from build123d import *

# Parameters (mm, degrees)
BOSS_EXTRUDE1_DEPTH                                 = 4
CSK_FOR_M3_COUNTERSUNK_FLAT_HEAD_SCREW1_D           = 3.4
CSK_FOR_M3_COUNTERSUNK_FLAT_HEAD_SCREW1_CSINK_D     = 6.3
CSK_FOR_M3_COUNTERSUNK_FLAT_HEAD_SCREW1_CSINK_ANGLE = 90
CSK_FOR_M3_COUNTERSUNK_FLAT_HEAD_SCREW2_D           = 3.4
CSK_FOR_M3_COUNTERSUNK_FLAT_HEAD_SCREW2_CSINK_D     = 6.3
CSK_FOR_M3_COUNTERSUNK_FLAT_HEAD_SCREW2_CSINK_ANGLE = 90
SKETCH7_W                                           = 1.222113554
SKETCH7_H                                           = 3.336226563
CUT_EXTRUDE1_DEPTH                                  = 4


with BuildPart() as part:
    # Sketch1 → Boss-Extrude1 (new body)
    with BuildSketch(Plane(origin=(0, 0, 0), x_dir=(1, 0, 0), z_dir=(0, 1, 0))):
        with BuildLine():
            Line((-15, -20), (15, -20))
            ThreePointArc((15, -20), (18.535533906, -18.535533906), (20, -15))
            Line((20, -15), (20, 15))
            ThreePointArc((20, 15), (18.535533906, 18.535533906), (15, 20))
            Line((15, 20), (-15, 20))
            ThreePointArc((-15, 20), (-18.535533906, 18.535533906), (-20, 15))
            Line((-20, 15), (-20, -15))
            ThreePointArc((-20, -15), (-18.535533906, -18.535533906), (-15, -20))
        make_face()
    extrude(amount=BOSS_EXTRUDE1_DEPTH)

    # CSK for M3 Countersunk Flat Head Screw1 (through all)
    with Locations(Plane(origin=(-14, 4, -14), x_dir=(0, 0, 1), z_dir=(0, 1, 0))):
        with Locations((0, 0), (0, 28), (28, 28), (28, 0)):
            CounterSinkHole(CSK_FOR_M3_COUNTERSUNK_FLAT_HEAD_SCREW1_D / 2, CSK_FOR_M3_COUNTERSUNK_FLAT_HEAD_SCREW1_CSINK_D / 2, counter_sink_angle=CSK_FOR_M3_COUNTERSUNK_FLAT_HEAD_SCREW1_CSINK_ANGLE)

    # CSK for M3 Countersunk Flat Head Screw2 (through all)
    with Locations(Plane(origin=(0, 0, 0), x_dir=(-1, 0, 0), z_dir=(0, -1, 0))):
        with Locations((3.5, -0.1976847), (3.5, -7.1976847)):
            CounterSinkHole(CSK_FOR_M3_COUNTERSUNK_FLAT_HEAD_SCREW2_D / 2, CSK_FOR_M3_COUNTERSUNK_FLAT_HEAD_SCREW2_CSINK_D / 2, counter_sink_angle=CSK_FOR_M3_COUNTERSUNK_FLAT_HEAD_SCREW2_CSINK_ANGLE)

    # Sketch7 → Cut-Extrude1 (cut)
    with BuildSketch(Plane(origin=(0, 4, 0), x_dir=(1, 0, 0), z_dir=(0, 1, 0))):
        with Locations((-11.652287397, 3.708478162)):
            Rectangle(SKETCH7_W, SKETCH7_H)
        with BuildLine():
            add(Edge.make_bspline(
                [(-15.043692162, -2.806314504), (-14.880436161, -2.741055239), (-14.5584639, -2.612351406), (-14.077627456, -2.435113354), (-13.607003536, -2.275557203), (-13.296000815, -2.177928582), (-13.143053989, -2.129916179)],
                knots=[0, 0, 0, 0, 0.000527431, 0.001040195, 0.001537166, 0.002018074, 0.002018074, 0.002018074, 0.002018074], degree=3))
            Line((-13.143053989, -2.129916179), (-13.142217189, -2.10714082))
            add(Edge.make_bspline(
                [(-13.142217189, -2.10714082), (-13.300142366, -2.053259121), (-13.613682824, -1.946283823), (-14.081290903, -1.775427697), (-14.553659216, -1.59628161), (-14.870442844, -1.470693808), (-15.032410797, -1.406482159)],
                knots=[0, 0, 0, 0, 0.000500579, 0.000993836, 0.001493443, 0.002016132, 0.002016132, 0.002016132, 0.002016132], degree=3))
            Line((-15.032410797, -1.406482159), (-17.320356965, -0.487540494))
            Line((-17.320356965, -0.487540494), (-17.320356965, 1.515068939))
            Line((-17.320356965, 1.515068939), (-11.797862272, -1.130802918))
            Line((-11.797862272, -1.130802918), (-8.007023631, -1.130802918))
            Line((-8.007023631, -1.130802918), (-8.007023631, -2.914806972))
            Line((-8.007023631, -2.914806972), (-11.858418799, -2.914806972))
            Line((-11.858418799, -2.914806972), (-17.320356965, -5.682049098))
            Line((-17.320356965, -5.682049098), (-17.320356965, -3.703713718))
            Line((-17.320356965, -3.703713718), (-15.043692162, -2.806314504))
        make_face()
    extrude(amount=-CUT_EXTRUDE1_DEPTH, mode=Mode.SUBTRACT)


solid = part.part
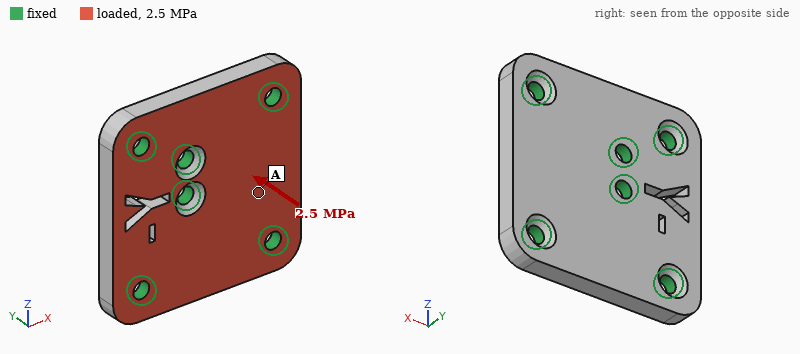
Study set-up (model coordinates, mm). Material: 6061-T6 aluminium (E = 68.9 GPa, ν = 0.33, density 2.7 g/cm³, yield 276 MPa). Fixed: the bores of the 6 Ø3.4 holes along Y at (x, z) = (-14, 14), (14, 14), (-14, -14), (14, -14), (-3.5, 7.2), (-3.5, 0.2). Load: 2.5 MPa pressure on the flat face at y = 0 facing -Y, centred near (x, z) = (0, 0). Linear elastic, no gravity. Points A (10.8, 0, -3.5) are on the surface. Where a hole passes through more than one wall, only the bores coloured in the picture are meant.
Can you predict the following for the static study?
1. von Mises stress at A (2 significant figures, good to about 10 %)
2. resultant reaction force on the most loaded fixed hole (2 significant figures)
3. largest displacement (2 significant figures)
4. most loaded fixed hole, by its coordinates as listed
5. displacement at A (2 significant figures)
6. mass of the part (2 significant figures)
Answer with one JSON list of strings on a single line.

["20 MPa", "790 N", "16 µm", "(14, -14)", "11 µm", "16 g"]
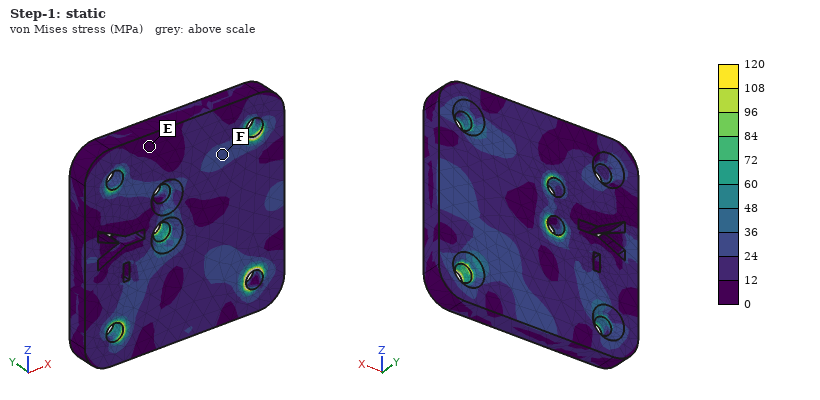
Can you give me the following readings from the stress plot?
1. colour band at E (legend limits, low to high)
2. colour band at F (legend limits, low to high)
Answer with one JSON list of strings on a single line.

["0 to 12 MPa", "24 to 36 MPa"]
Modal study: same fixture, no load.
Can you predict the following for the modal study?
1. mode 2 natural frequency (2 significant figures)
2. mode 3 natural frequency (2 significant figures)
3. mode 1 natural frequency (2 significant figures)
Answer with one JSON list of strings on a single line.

["23 kHz", "26 kHz", "22 kHz"]
